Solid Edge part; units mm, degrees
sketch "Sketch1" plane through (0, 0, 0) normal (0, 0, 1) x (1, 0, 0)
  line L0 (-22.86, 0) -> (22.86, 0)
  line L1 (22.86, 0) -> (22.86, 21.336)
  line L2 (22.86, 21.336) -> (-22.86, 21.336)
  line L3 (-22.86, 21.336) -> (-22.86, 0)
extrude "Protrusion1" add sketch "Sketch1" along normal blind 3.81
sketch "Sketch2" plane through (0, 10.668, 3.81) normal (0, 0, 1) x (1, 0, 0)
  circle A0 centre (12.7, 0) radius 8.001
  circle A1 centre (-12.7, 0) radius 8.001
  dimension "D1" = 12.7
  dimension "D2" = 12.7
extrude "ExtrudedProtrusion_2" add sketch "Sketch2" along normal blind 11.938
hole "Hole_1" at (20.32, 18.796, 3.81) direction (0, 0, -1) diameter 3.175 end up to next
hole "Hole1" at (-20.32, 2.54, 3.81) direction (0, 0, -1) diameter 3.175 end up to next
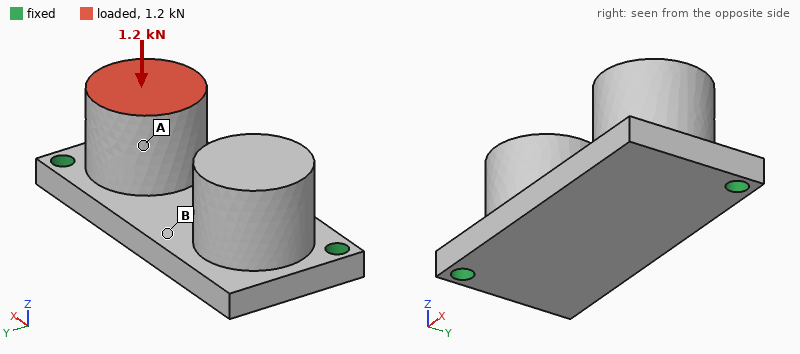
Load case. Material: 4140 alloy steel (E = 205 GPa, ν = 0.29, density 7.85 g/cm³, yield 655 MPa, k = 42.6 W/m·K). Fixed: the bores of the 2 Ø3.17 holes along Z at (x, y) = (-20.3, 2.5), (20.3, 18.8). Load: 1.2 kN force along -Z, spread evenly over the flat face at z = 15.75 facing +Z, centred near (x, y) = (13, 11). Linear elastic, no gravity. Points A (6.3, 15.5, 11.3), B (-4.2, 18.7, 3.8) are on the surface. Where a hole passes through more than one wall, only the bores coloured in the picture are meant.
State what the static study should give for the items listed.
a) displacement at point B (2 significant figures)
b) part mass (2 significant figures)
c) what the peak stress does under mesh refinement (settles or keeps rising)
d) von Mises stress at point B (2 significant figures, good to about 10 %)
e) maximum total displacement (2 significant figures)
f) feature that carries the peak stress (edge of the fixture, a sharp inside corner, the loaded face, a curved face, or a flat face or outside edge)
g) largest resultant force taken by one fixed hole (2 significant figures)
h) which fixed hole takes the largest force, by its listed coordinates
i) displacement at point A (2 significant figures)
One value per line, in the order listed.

7.9 µm
66 g
keeps rising
40 MPa
34 µm
edge of the fixture
960 N
(20.3, 18.8)
18 µm
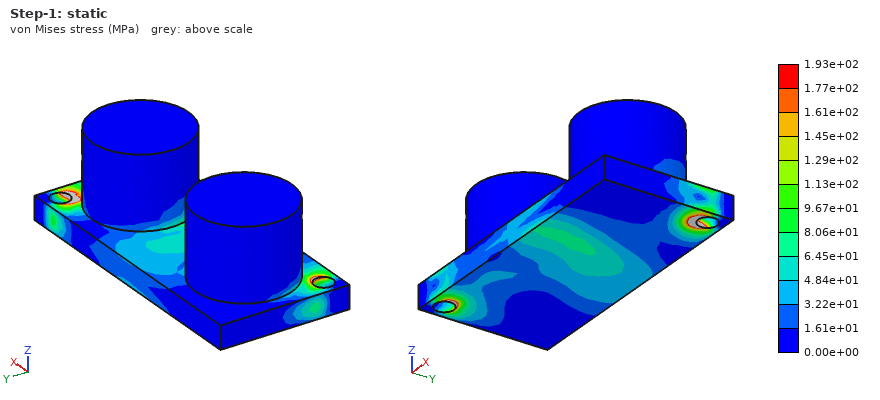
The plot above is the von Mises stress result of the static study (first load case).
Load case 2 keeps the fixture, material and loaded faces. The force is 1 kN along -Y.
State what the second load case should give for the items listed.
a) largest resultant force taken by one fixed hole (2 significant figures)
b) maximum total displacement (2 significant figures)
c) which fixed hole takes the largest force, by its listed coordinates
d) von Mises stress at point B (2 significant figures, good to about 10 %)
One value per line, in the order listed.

850 N
64 µm
(20.3, 18.8)
49 MPa
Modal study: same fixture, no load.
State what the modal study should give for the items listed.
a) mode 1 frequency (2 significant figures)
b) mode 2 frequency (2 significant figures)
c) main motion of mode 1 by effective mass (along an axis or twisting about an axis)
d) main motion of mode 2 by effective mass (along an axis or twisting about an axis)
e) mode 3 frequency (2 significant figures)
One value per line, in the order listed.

5000 Hz
5200 Hz
along Y
along Z
9000 Hz
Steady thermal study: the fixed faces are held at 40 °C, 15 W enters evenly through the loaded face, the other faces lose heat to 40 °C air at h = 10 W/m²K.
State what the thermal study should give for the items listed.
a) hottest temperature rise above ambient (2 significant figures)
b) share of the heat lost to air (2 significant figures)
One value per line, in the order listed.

57 K
5.6 %
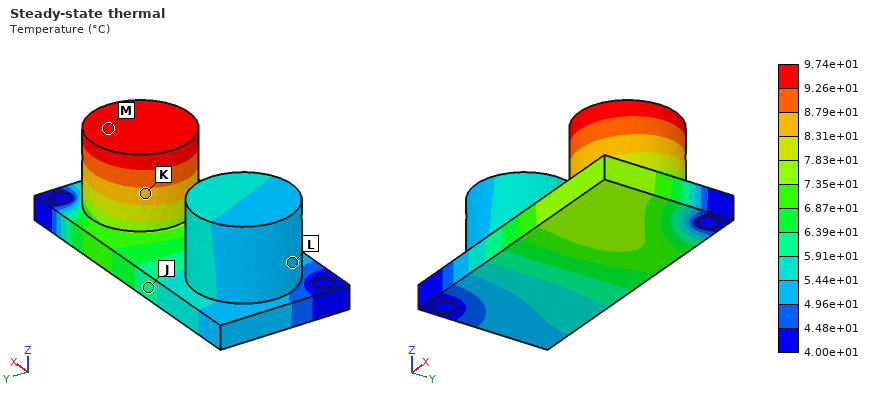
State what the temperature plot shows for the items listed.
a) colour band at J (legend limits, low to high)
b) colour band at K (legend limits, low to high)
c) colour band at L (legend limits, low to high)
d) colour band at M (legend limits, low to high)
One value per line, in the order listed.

5.91e+01 to 6.39e+01 °C
8.31e+01 to 8.79e+01 °C
4.96e+01 to 5.44e+01 °C
9.26e+01 to 9.74e+01 °C
